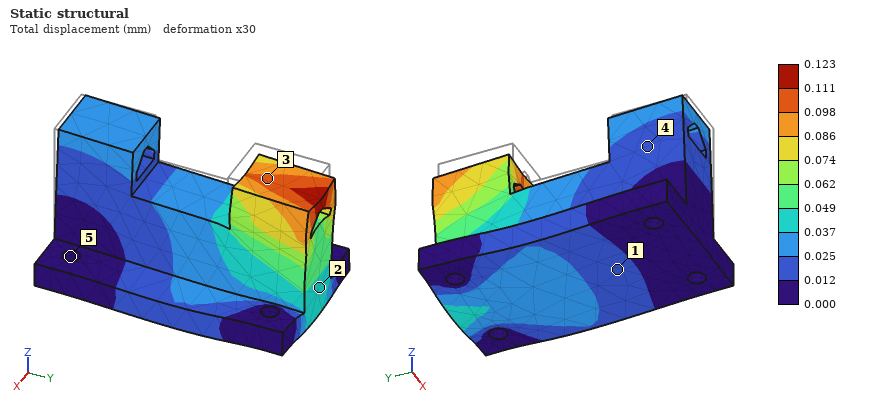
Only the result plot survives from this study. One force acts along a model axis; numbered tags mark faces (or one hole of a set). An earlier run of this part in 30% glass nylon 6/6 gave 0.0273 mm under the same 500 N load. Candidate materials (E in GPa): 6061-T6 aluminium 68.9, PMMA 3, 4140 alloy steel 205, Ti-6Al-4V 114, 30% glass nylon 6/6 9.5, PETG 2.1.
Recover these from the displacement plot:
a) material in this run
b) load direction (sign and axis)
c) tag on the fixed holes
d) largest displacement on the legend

PETG
-Z
5
0.123 mm
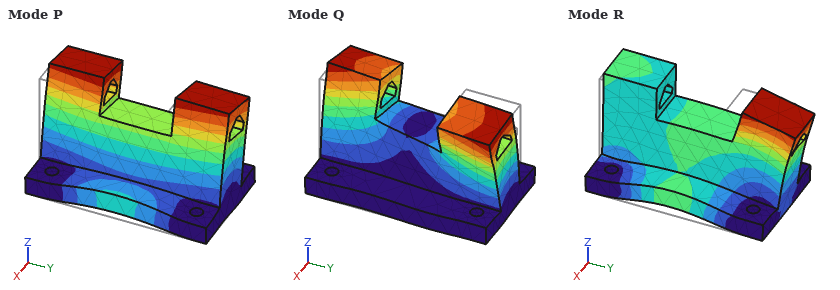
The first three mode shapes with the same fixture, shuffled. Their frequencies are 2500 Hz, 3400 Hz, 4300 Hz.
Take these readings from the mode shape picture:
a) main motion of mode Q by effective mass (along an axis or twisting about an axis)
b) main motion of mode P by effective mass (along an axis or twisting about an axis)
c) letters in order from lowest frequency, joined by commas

twisting about Z
along X
P, Q, R
